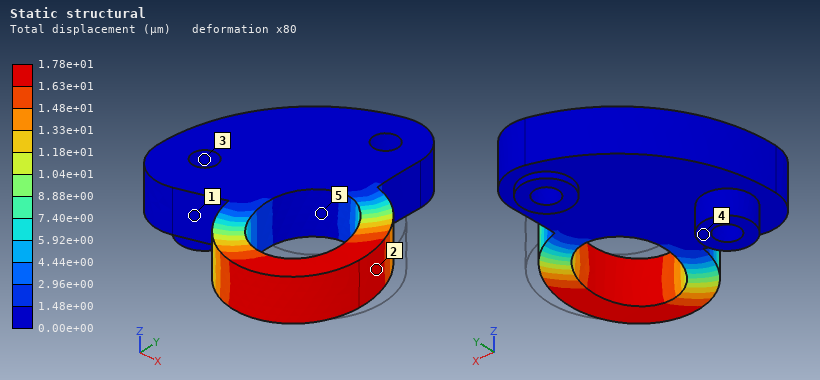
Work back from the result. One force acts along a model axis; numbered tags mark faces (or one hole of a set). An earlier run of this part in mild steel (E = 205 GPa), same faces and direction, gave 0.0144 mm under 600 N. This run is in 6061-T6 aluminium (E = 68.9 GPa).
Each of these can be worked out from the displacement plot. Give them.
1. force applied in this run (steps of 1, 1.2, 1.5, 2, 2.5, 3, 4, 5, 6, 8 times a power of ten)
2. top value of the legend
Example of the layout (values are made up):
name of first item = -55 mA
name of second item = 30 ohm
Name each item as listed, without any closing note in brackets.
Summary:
force applied in this run = 250 N
top value of the legend = 1.78e+01 µm
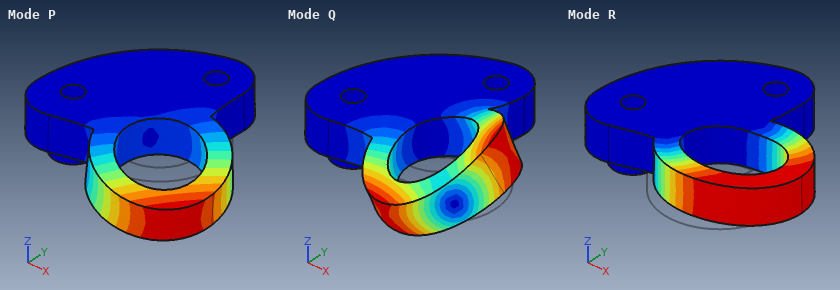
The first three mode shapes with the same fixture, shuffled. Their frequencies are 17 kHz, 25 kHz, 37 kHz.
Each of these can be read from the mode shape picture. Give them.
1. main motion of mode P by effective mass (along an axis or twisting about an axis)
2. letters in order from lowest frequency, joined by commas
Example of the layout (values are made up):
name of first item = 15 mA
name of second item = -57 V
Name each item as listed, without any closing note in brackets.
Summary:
main motion of mode P by effective mass = along Z
letters in order from lowest frequency, joined by commas = P, R, Q
